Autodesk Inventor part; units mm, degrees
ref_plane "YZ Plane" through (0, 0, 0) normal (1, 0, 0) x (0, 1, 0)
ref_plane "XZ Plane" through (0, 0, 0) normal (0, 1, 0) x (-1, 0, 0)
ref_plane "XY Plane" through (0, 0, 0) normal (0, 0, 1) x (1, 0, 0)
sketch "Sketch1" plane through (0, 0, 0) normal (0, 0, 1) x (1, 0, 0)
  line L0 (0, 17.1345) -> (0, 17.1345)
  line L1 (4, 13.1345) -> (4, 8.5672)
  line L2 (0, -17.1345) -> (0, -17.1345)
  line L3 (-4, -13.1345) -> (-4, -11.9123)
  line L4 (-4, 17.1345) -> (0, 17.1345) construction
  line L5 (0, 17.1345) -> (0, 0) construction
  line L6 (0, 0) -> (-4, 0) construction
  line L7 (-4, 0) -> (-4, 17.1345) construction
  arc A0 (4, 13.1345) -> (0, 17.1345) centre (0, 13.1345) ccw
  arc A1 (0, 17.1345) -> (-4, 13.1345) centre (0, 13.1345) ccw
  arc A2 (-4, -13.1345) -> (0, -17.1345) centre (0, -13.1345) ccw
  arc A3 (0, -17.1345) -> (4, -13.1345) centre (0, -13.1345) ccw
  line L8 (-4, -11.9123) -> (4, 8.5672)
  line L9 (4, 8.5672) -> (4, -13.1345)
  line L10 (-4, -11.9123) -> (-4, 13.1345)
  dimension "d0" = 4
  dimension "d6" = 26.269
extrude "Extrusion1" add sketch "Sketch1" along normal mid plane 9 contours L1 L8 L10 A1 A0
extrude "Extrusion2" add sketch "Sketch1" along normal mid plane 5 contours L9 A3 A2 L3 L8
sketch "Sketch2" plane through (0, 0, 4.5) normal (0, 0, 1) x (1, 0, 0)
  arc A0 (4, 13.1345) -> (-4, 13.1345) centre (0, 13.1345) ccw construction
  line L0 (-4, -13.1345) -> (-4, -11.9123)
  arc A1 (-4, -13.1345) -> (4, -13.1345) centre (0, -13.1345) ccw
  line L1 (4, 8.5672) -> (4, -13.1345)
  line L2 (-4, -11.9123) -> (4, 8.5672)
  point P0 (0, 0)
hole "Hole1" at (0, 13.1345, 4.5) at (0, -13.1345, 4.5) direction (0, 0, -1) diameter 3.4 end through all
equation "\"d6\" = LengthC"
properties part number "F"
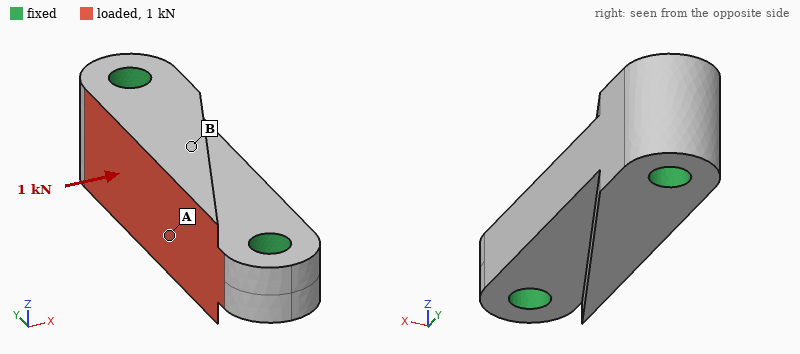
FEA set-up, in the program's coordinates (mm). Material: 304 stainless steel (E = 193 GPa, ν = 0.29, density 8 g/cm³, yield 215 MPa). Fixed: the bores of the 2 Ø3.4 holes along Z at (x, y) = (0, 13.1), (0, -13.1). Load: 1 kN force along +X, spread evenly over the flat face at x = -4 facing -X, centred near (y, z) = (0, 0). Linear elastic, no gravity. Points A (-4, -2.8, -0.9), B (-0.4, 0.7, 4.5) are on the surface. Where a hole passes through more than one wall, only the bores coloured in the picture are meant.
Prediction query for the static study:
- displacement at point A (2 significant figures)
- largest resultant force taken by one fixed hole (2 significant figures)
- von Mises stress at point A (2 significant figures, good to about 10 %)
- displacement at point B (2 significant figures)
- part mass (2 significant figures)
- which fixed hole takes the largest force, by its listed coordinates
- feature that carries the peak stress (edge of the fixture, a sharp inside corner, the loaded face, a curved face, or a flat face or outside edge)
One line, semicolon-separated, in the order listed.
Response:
1.9 µm; 550 N; 21 MPa; 2.0 µm; 14 g; (0, 13.1); the loaded face
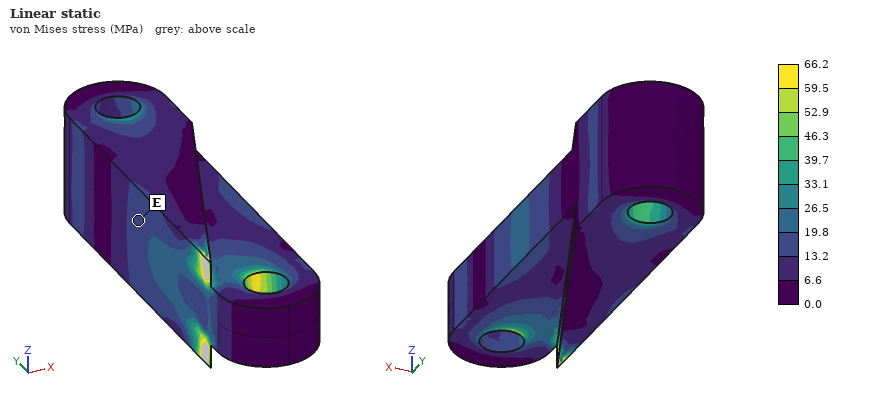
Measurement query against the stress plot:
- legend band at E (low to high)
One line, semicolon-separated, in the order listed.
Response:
13.2 to 19.8 MPa
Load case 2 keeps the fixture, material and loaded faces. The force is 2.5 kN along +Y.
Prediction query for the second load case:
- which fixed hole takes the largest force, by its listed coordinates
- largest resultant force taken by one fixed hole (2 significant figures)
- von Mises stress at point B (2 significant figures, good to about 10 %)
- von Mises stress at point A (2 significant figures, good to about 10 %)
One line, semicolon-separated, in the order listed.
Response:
(0, 13.1); 1.5 kN; 9.2 MPa; 21 MPa
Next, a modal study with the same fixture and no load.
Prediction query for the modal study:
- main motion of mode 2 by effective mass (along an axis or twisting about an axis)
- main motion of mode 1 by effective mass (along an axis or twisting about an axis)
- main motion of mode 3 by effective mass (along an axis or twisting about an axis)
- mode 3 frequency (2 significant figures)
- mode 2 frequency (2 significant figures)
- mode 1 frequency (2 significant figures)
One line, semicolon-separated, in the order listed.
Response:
along Z; along X; twisting about Y; 53 kHz; 40 kHz; 37 kHz
